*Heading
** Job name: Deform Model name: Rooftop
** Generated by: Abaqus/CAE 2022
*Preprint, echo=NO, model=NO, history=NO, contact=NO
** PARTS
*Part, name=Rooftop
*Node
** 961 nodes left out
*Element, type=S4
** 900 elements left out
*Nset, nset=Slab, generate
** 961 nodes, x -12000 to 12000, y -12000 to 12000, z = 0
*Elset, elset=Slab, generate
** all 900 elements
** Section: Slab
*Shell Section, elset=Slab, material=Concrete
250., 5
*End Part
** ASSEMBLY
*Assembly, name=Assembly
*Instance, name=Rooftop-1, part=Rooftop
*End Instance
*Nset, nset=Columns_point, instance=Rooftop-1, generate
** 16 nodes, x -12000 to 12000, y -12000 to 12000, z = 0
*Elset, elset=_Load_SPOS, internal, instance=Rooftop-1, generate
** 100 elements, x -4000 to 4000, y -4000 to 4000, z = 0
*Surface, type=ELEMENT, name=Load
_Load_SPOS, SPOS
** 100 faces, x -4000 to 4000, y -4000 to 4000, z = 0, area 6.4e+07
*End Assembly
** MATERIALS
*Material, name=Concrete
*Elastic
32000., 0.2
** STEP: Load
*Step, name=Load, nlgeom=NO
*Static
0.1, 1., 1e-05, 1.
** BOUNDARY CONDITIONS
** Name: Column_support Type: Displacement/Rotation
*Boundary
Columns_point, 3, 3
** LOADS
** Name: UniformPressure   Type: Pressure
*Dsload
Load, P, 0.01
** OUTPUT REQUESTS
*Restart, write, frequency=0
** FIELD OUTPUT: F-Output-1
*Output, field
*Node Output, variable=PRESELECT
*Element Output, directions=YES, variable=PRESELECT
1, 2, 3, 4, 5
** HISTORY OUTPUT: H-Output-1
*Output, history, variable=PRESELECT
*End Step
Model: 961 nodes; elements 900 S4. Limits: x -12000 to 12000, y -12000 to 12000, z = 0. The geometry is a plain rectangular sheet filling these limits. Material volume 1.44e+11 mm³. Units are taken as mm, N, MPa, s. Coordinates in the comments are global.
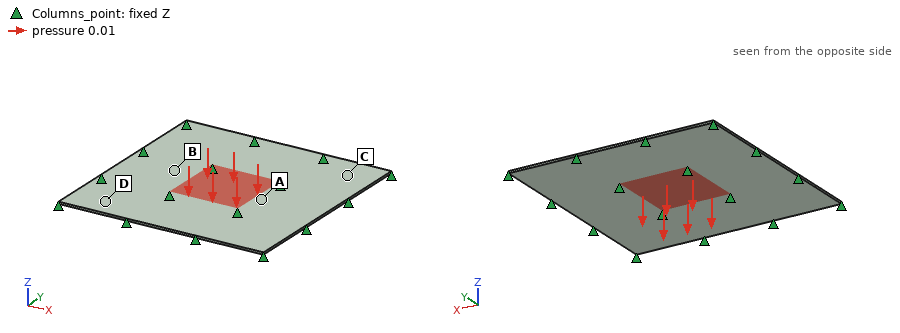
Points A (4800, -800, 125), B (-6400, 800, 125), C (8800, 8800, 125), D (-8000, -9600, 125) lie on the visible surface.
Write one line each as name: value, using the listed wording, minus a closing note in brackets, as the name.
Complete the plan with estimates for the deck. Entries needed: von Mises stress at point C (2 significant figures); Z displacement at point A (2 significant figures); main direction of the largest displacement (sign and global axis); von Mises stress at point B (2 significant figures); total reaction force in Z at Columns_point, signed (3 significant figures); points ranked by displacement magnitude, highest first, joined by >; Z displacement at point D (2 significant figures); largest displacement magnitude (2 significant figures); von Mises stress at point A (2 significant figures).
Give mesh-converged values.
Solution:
von Mises stress at point C: 0.33 MPa
Z displacement at point A: -2.4 mm
main direction of the largest displacement: -Z
von Mises stress at point B: 1.9 MPa
total reaction force in Z at Columns_point, signed: 6.40e+05 N
points ranked by displacement magnitude, highest first, joined by >: A > C > D > B
Z displacement at point D: 1.1 mm
largest displacement magnitude: 7.8 mm
von Mises stress at point A: 2.4 MPa
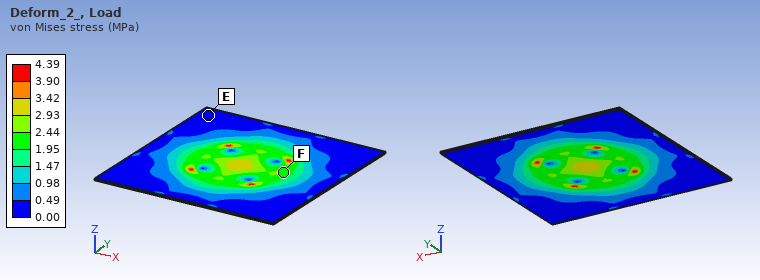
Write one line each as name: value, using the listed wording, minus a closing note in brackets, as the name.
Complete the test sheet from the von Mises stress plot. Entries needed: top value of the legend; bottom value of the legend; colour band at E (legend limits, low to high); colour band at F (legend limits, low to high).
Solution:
top value of the legend: 4.39 MPa
bottom value of the legend: 0.00 MPa
colour band at E: 0.00 to 0.49 MPa
colour band at F: 1.95 to 2.44 MPa
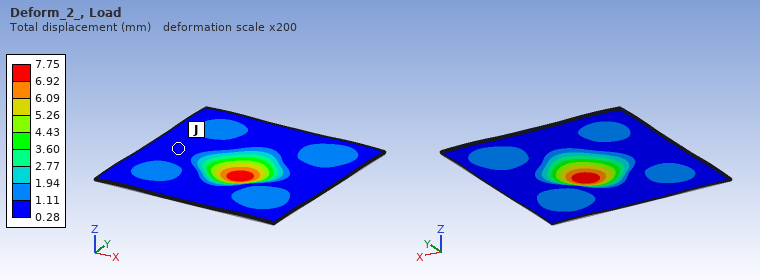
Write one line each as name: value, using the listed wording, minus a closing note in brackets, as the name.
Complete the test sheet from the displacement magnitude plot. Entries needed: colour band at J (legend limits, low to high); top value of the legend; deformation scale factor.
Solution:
colour band at J: 0.28 to 1.11 mm
top value of the legend: 7.75 mm
deformation scale factor: 200
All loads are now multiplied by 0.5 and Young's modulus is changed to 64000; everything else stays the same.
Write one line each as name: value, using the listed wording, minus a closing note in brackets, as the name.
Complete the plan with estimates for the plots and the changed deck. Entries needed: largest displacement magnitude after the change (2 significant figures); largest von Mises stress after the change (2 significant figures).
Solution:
largest displacement magnitude after the change: 1.9 mm
largest von Mises stress after the change: 2.2 MPa
